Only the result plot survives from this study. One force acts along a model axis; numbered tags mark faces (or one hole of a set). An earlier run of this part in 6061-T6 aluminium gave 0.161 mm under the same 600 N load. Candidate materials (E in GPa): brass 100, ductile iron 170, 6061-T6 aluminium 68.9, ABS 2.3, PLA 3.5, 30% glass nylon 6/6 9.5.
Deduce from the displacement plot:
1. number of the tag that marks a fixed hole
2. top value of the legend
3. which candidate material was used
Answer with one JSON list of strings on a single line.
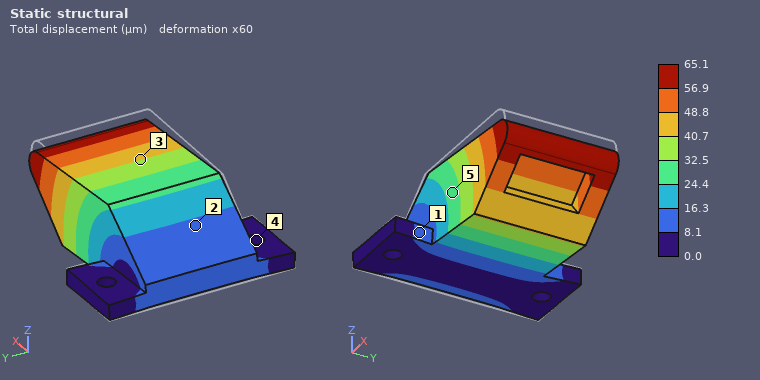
["4", "65.1 µm", "ductile iron"]
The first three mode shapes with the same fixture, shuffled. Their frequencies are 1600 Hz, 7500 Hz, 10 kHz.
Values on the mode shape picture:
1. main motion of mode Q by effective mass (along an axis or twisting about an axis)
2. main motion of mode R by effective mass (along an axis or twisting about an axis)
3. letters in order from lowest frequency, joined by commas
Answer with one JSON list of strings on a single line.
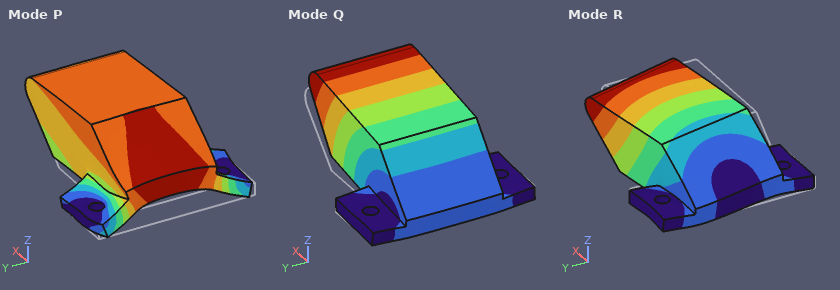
["along Z", "along Y", "Q, R, P"]
